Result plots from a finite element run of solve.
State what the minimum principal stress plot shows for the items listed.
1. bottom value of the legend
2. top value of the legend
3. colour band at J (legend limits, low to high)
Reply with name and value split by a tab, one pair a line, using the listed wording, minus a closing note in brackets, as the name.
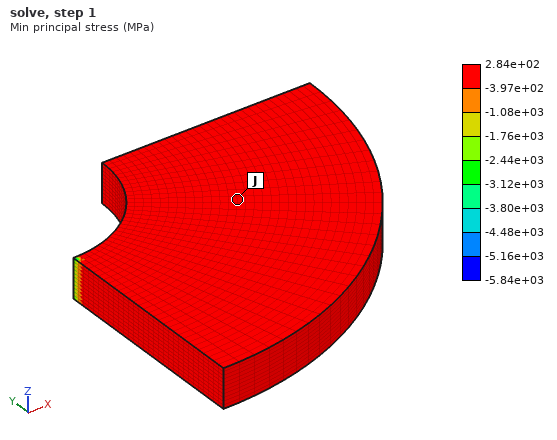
bottom value of the legend	-5.84e+03 MPa
top value of the legend	2.84e+02 MPa
colour band at J	-3.97e+02 to 2.84e+02 MPa
